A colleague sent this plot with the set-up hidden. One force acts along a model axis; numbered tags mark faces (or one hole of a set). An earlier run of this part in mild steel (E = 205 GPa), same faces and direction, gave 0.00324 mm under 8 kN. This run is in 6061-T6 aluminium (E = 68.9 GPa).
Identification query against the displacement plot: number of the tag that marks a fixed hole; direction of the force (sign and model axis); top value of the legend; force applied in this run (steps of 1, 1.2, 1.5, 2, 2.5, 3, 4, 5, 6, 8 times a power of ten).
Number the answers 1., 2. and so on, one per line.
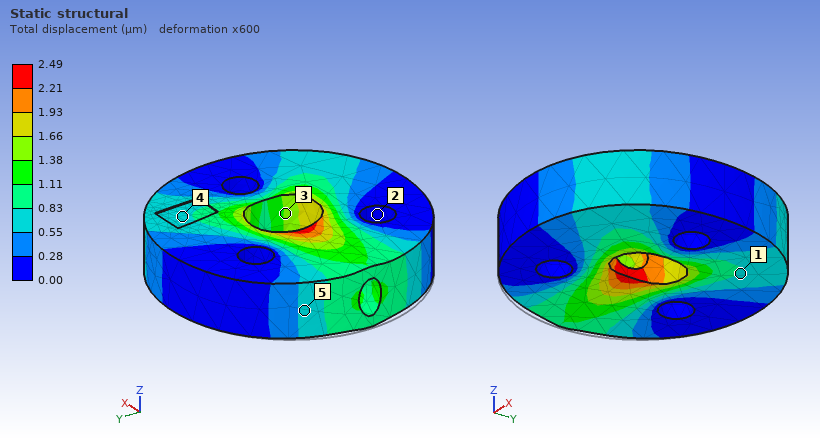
1. 2
2. +X
3. 2.49 µm
4. 2 kN
